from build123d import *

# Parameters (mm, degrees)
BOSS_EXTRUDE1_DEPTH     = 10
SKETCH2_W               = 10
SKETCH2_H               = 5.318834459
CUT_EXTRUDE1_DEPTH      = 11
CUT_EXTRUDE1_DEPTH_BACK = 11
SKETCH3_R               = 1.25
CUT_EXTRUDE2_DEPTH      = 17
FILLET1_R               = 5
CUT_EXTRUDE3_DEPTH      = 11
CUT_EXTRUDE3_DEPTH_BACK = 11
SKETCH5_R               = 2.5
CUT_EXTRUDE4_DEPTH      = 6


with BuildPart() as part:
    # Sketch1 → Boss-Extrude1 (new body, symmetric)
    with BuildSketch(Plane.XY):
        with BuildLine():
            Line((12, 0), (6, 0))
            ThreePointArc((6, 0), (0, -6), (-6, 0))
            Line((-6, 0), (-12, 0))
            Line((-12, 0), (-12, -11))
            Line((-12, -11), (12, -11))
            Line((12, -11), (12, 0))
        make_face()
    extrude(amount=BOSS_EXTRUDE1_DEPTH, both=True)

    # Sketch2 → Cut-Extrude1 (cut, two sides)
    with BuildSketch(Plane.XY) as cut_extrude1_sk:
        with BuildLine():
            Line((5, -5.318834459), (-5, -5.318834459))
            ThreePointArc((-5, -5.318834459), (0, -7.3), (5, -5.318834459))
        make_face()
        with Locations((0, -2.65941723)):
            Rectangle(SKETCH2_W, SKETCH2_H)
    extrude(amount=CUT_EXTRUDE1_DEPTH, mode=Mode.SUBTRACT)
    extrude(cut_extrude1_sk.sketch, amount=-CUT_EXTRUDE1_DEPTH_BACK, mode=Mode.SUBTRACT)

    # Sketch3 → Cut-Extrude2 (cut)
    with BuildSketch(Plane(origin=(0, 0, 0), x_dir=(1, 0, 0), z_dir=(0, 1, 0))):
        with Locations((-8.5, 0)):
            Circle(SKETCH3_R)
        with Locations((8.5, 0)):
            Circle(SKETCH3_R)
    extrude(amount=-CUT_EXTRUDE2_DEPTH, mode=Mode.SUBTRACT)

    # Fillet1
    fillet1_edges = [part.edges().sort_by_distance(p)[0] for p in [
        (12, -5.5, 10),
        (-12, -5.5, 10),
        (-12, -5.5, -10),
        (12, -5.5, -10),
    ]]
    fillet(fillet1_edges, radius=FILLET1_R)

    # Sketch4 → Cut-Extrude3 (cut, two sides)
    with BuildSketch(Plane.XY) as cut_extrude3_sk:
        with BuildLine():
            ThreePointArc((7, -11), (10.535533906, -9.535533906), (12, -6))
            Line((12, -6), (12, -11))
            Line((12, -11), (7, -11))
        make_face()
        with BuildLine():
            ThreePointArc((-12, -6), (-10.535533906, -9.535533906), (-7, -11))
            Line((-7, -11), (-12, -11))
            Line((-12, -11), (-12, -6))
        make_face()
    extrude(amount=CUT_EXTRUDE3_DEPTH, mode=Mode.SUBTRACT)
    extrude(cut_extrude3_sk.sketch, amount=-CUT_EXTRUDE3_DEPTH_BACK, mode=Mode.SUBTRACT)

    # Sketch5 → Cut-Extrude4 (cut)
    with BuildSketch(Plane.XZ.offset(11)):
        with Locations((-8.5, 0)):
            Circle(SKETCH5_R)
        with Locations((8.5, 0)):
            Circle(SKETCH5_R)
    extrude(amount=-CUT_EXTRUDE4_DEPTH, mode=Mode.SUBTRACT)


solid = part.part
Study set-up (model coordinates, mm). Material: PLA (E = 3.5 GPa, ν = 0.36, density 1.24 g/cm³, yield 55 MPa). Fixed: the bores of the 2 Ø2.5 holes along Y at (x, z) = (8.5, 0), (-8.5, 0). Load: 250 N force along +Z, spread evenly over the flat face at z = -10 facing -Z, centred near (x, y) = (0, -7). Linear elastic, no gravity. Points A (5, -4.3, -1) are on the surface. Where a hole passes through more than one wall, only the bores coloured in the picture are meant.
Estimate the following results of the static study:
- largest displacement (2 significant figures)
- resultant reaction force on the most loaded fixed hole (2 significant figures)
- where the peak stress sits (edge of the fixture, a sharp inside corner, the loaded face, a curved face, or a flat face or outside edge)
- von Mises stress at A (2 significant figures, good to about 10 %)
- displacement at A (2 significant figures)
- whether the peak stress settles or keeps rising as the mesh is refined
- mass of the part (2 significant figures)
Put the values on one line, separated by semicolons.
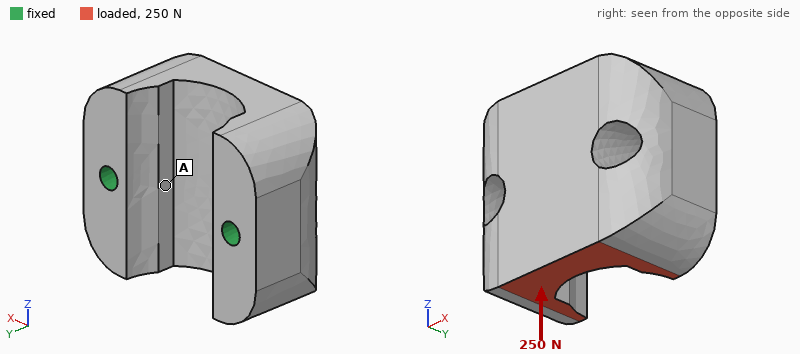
68 µm; 130 N; edge of the fixture; 3.7 MPa; 10 µm; keeps rising; 3.9 g
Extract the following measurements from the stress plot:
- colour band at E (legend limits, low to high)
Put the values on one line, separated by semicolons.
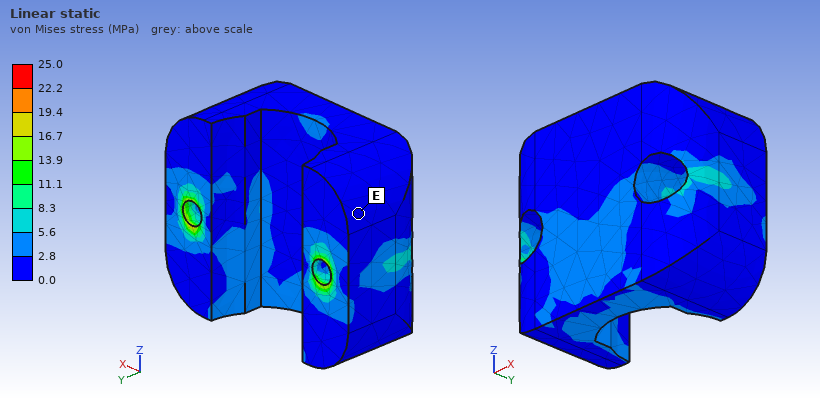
0.0 to 2.8 MPa
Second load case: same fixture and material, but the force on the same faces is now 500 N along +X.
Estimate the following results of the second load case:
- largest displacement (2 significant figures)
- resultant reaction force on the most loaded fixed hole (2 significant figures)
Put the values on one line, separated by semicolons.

0.12 mm; 340 N
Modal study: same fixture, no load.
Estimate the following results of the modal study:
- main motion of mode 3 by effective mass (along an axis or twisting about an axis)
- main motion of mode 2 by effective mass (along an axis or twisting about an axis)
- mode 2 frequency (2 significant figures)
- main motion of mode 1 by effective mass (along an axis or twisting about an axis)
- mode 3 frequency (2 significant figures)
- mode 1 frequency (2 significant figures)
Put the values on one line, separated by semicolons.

along X; twisting about Y; 9500 Hz; along Z; 12 kHz; 6200 Hz
